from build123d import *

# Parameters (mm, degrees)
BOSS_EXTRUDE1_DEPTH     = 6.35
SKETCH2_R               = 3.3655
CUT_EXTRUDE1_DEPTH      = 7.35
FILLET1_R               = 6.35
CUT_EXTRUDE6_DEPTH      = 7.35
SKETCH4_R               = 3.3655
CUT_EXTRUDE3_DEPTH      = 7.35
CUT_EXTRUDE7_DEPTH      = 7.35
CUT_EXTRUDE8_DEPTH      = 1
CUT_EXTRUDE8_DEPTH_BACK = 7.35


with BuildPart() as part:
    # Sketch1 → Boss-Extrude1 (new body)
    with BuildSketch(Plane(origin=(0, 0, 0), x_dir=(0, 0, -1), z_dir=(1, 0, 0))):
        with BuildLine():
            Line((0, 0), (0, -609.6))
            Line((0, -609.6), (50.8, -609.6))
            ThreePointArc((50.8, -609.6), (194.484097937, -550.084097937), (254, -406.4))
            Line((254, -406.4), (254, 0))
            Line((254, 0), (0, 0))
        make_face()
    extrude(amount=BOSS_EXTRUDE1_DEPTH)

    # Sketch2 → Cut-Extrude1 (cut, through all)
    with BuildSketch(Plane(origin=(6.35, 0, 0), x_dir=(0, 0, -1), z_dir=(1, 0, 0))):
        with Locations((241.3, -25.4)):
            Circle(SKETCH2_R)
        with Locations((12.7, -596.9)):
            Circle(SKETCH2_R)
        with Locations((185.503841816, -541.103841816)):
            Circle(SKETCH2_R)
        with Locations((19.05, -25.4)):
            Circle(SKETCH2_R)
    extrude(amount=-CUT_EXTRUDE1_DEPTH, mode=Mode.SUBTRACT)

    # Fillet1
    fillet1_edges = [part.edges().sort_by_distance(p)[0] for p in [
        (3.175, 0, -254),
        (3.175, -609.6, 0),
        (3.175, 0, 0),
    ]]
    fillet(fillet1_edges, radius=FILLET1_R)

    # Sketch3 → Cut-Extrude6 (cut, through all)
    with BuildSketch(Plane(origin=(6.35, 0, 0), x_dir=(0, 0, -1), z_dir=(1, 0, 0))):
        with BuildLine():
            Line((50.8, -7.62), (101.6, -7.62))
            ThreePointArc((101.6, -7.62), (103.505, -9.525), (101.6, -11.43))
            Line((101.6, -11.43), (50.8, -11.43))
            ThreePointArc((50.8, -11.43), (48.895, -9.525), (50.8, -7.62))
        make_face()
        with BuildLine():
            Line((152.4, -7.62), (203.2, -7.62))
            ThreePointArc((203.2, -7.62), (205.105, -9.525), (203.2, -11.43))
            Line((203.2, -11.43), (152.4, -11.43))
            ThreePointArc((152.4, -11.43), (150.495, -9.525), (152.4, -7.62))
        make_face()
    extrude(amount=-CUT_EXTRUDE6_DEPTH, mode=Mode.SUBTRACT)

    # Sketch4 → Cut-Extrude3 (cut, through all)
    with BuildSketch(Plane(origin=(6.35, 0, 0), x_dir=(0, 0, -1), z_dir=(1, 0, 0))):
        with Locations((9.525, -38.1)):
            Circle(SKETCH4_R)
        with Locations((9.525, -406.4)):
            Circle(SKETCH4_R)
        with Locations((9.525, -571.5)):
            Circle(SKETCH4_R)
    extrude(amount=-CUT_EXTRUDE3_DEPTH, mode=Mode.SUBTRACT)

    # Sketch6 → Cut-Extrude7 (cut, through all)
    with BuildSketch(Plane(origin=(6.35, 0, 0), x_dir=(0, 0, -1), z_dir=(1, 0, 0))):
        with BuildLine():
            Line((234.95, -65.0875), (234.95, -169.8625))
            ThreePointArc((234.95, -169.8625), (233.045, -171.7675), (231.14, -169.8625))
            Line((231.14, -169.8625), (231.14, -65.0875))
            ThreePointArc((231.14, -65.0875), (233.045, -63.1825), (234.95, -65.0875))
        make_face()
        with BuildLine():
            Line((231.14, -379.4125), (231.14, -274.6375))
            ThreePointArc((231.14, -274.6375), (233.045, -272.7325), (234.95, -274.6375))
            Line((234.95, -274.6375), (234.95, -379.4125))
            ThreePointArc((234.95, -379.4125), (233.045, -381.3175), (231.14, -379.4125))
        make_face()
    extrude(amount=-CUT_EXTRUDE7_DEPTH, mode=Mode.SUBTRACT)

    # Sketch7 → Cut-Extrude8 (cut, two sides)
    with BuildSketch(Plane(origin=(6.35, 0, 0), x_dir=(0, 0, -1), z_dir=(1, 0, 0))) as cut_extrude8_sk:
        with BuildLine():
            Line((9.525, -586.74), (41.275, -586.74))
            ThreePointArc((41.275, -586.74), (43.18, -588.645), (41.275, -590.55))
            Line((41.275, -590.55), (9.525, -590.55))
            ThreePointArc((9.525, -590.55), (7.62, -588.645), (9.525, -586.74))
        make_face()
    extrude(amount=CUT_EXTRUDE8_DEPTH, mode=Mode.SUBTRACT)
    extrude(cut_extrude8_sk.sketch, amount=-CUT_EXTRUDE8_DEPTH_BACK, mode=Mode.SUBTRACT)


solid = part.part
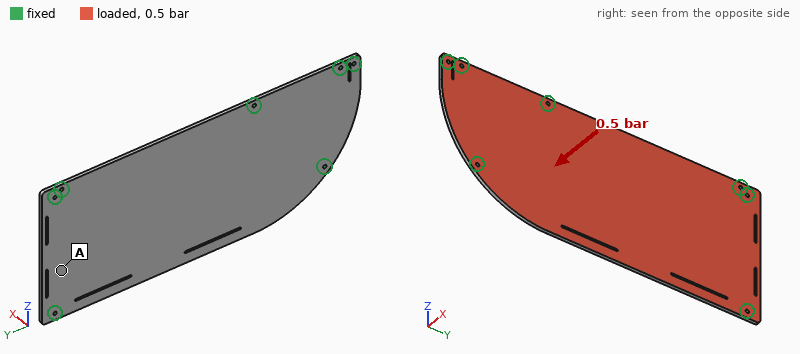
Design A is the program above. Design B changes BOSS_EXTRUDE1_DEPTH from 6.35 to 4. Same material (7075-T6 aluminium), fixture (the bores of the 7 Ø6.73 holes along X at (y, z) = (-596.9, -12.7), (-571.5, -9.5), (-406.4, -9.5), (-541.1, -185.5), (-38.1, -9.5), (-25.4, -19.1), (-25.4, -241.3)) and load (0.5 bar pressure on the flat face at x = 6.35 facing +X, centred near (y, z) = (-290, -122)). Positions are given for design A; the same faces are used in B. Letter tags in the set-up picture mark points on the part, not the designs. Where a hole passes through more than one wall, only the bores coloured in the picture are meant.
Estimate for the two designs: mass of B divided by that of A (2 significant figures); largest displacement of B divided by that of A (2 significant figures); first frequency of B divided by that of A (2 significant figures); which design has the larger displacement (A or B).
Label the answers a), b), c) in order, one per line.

a) 0.63
b) 3.9
c) 0.64
d) B
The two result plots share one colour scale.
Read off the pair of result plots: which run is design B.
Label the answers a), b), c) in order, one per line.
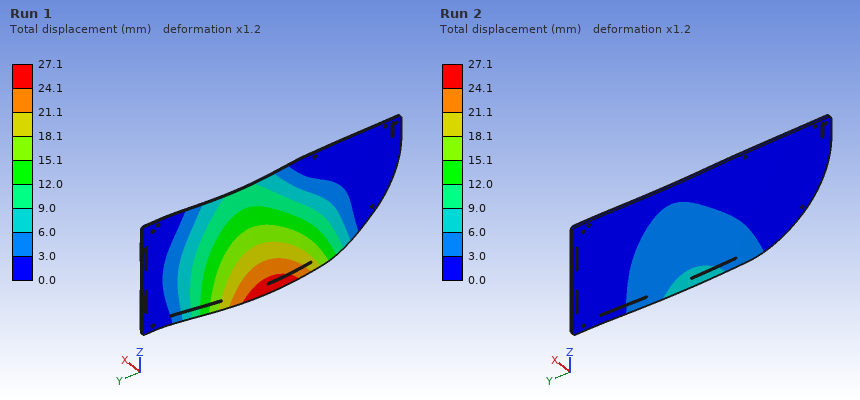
a) Run 1
